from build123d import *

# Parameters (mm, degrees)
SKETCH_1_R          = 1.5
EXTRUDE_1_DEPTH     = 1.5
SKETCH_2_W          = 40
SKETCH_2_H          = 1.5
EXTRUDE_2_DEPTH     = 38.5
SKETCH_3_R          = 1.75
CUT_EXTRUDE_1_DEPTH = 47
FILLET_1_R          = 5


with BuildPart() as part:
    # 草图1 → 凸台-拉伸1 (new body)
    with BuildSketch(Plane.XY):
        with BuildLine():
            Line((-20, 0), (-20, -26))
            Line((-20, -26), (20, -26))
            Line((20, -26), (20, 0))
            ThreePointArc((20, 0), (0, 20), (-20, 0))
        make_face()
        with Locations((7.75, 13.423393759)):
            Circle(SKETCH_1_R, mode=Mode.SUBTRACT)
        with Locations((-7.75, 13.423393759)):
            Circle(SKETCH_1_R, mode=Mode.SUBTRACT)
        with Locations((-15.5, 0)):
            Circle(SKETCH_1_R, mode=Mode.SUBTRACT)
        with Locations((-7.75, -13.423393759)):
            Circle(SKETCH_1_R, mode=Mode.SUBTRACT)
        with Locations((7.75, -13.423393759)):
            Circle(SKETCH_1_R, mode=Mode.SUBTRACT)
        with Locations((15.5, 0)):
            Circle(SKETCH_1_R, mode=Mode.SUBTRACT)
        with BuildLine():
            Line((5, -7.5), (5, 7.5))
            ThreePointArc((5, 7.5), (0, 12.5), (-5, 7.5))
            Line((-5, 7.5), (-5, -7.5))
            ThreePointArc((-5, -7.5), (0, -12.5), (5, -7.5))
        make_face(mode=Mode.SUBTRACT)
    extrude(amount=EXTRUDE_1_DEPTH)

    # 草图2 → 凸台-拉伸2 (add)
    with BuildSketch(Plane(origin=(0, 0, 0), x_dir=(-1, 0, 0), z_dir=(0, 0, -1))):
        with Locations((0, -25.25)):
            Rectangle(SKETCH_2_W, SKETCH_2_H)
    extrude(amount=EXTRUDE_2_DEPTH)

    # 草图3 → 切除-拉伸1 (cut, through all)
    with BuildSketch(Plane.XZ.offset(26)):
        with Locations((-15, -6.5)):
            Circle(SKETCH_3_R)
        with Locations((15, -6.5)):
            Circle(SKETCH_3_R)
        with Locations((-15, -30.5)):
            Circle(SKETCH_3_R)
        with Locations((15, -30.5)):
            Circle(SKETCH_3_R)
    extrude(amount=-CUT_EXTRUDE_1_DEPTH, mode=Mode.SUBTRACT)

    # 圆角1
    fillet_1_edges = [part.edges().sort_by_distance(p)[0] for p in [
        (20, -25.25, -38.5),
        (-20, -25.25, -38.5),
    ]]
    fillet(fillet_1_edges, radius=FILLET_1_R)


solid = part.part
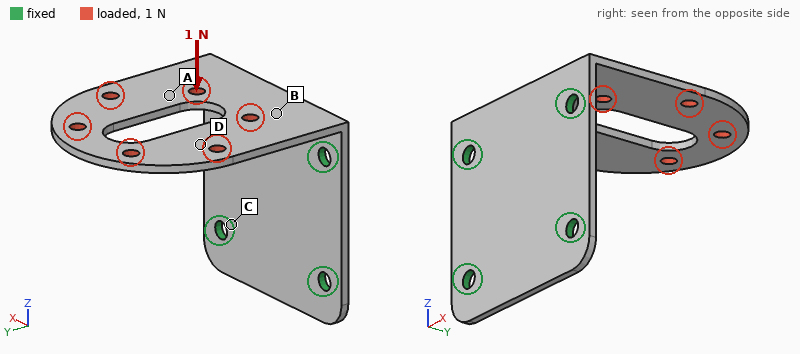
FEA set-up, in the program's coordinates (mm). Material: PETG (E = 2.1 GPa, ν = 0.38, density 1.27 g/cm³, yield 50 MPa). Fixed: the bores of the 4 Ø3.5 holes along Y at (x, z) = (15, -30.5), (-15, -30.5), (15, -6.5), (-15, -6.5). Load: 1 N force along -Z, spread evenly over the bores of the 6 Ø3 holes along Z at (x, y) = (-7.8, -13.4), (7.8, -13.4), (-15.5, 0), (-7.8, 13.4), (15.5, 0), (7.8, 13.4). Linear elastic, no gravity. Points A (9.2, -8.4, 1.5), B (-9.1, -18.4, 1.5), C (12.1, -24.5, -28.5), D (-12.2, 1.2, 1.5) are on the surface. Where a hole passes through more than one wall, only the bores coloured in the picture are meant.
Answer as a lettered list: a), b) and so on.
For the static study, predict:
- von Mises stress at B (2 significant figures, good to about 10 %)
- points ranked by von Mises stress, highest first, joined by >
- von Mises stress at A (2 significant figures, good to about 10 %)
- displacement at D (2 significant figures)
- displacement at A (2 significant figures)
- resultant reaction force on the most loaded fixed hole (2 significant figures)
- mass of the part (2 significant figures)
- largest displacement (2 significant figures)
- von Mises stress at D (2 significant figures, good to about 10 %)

a) 1.0 MPa
b) B > A > D > C
c) 0.85 MPa
d) 0.42 mm
e) 0.22 mm
f) 0.34 N
g) 5.5 g
h) 0.87 mm
i) 0.46 MPa
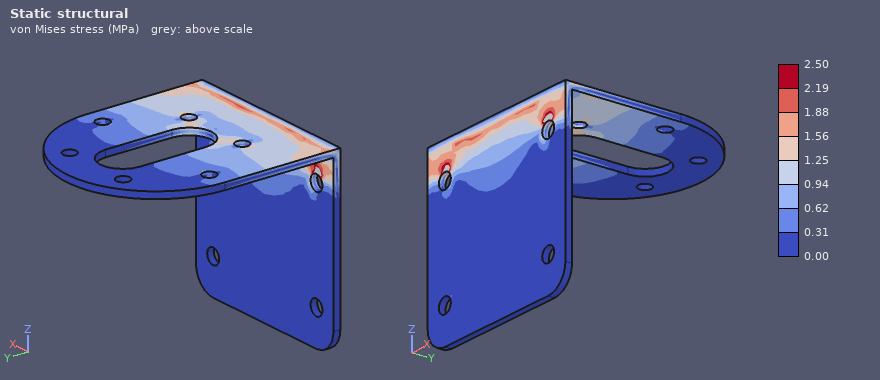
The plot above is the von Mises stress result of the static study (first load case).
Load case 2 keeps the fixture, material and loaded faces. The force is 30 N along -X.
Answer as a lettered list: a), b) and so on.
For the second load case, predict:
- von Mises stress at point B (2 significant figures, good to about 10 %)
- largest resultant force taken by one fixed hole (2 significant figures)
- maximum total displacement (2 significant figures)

a) 2.0 MPa
b) 30 N
c) 0.76 mm
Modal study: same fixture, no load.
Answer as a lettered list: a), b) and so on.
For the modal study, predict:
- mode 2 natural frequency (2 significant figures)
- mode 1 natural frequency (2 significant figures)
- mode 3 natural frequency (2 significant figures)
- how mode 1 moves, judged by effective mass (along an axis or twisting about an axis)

a) 430 Hz
b) 160 Hz
c) 820 Hz
d) along Z
